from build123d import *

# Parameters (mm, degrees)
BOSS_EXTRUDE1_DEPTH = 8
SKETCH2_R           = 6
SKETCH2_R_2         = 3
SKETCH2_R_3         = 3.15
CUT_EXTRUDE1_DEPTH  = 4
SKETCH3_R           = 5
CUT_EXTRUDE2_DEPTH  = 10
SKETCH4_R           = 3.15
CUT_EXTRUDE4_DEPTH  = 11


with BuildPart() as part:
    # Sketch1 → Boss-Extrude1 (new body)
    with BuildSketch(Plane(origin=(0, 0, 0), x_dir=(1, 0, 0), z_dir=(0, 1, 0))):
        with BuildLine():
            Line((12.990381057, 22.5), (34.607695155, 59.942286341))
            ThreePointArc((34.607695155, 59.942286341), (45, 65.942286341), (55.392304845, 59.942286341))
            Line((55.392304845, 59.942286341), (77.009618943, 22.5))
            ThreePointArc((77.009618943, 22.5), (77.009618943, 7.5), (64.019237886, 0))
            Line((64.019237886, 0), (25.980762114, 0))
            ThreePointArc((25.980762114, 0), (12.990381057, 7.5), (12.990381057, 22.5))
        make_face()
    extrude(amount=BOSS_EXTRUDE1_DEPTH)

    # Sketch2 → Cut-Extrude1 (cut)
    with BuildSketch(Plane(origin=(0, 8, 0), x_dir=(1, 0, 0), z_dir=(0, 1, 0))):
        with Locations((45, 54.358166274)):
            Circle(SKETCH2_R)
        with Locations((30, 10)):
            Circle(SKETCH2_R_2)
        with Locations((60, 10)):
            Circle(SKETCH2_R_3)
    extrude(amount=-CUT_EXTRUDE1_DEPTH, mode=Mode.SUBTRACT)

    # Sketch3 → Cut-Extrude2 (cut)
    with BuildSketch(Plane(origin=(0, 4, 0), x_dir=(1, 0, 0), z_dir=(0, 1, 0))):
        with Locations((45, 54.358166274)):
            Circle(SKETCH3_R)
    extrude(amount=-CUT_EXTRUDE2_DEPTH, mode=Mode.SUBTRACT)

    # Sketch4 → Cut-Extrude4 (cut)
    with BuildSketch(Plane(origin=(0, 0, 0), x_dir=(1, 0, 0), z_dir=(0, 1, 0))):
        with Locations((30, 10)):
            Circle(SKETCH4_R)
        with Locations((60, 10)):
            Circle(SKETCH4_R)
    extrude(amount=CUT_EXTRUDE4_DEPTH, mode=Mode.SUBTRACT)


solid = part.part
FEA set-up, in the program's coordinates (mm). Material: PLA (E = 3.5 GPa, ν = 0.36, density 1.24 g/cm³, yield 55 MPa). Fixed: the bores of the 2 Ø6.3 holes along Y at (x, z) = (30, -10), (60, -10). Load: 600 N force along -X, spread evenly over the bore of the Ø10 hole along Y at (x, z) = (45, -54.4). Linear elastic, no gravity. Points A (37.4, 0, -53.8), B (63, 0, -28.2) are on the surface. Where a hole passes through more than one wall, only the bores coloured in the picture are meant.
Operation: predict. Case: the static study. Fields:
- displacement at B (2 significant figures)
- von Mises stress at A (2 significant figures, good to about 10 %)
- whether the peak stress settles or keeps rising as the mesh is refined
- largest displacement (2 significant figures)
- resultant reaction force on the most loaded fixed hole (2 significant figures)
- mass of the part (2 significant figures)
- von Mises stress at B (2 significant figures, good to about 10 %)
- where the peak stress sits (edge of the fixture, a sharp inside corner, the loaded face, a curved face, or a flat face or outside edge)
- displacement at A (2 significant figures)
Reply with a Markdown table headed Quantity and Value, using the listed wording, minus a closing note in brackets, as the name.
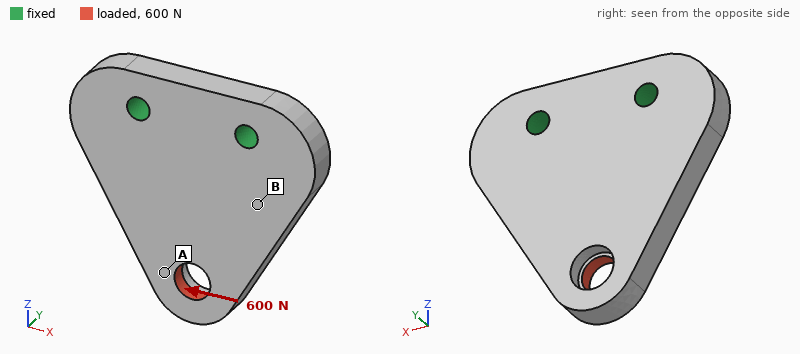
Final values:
| Quantity | Value |
|---|---|
| displacement at B | 0.053 mm |
| von Mises stress at A | 11 MPa |
| whether the peak stress settles or keeps rising as the mesh is refined | keeps rising |
| largest displacement | 0.20 mm |
| resultant reaction force on the most loaded fixed hole | 820 N |
| mass of the part | 29 g |
| von Mises stress at B | 3.5 MPa |
| where the peak stress sits | edge of the fixture |
| displacement at A | 0.15 mm |
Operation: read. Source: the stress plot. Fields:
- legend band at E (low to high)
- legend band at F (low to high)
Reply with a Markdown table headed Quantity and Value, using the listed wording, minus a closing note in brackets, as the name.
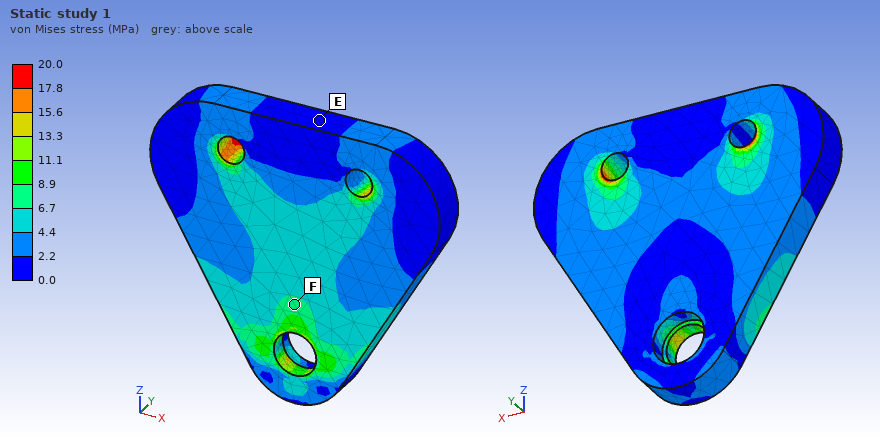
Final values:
| Quantity | Value |
|---|---|
| legend band at E | 0.0 to 2.2 MPa |
| legend band at F | 6.7 to 8.9 MPa |
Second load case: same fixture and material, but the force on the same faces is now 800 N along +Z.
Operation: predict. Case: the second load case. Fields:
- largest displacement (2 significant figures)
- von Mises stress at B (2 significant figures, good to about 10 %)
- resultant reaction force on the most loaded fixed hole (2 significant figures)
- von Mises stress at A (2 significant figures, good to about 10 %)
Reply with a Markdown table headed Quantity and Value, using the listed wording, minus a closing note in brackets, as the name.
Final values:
| Quantity | Value |
|---|---|
| largest displacement | 0.37 mm |
| von Mises stress at B | 4.5 MPa |
| resultant reaction force on the most loaded fixed hole | 410 N |
| von Mises stress at A | 8.2 MPa |
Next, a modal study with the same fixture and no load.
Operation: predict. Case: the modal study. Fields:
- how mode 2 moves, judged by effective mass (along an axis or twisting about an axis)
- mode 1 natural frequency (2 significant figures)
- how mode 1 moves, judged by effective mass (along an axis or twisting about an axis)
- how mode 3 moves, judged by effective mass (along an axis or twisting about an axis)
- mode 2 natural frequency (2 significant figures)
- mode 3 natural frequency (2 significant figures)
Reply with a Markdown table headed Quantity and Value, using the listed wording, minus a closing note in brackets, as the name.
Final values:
| Quantity | Value |
|---|---|
| how mode 2 moves, judged by effective mass | twisting about Z |
| mode 1 natural frequency | 1100 Hz |
| how mode 1 moves, judged by effective mass | along Y |
| how mode 3 moves, judged by effective mass | along X |
| mode 2 natural frequency | 3000 Hz |
| mode 3 natural frequency | 3800 Hz |
